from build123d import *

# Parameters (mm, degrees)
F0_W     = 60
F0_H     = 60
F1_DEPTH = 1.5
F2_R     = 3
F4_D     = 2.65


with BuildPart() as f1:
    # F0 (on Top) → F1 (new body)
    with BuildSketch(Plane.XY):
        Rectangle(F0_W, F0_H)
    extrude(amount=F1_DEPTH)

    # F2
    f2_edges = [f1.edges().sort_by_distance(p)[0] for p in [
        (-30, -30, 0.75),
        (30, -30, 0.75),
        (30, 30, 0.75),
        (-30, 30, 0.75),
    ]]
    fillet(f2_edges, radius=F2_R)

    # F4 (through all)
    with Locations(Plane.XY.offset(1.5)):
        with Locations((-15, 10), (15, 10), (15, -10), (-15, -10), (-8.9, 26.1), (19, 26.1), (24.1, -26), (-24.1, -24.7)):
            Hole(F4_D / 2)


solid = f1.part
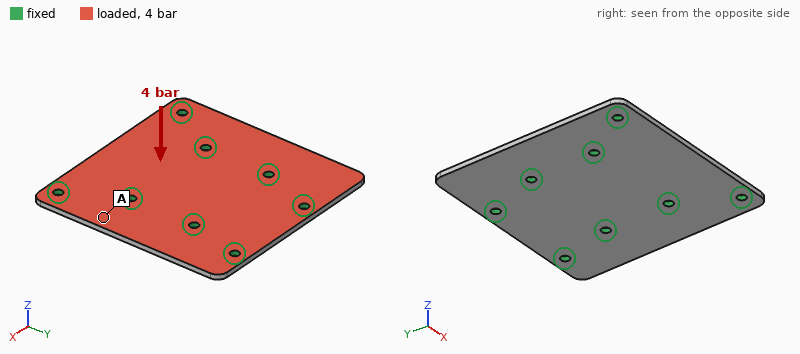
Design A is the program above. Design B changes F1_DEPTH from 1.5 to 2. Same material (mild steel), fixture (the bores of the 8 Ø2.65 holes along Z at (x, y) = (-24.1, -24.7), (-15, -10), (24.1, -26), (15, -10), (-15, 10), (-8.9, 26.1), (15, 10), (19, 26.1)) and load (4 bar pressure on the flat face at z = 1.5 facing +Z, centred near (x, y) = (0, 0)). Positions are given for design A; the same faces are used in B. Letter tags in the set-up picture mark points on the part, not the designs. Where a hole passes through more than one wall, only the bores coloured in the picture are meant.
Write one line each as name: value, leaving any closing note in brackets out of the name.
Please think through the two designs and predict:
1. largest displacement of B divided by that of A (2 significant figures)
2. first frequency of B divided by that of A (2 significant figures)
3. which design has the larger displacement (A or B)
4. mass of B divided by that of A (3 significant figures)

largest displacement of B divided by that of A: 0.43
first frequency of B divided by that of A: 1.3
which design has the larger displacement: A
mass of B divided by that of A: 1.33
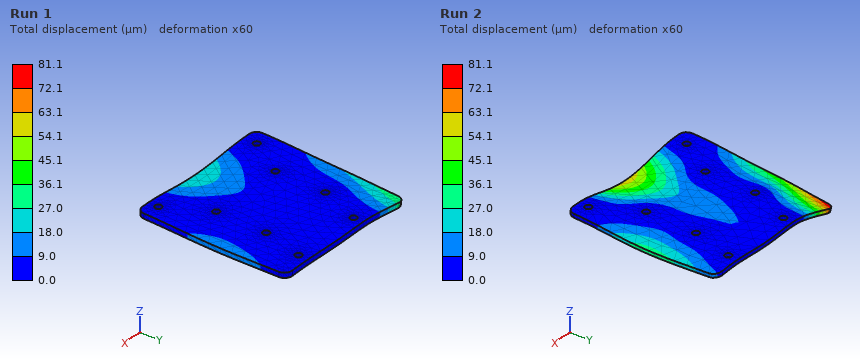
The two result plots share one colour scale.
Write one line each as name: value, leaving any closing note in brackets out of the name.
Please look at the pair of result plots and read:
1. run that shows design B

run that shows design B: Run 1
